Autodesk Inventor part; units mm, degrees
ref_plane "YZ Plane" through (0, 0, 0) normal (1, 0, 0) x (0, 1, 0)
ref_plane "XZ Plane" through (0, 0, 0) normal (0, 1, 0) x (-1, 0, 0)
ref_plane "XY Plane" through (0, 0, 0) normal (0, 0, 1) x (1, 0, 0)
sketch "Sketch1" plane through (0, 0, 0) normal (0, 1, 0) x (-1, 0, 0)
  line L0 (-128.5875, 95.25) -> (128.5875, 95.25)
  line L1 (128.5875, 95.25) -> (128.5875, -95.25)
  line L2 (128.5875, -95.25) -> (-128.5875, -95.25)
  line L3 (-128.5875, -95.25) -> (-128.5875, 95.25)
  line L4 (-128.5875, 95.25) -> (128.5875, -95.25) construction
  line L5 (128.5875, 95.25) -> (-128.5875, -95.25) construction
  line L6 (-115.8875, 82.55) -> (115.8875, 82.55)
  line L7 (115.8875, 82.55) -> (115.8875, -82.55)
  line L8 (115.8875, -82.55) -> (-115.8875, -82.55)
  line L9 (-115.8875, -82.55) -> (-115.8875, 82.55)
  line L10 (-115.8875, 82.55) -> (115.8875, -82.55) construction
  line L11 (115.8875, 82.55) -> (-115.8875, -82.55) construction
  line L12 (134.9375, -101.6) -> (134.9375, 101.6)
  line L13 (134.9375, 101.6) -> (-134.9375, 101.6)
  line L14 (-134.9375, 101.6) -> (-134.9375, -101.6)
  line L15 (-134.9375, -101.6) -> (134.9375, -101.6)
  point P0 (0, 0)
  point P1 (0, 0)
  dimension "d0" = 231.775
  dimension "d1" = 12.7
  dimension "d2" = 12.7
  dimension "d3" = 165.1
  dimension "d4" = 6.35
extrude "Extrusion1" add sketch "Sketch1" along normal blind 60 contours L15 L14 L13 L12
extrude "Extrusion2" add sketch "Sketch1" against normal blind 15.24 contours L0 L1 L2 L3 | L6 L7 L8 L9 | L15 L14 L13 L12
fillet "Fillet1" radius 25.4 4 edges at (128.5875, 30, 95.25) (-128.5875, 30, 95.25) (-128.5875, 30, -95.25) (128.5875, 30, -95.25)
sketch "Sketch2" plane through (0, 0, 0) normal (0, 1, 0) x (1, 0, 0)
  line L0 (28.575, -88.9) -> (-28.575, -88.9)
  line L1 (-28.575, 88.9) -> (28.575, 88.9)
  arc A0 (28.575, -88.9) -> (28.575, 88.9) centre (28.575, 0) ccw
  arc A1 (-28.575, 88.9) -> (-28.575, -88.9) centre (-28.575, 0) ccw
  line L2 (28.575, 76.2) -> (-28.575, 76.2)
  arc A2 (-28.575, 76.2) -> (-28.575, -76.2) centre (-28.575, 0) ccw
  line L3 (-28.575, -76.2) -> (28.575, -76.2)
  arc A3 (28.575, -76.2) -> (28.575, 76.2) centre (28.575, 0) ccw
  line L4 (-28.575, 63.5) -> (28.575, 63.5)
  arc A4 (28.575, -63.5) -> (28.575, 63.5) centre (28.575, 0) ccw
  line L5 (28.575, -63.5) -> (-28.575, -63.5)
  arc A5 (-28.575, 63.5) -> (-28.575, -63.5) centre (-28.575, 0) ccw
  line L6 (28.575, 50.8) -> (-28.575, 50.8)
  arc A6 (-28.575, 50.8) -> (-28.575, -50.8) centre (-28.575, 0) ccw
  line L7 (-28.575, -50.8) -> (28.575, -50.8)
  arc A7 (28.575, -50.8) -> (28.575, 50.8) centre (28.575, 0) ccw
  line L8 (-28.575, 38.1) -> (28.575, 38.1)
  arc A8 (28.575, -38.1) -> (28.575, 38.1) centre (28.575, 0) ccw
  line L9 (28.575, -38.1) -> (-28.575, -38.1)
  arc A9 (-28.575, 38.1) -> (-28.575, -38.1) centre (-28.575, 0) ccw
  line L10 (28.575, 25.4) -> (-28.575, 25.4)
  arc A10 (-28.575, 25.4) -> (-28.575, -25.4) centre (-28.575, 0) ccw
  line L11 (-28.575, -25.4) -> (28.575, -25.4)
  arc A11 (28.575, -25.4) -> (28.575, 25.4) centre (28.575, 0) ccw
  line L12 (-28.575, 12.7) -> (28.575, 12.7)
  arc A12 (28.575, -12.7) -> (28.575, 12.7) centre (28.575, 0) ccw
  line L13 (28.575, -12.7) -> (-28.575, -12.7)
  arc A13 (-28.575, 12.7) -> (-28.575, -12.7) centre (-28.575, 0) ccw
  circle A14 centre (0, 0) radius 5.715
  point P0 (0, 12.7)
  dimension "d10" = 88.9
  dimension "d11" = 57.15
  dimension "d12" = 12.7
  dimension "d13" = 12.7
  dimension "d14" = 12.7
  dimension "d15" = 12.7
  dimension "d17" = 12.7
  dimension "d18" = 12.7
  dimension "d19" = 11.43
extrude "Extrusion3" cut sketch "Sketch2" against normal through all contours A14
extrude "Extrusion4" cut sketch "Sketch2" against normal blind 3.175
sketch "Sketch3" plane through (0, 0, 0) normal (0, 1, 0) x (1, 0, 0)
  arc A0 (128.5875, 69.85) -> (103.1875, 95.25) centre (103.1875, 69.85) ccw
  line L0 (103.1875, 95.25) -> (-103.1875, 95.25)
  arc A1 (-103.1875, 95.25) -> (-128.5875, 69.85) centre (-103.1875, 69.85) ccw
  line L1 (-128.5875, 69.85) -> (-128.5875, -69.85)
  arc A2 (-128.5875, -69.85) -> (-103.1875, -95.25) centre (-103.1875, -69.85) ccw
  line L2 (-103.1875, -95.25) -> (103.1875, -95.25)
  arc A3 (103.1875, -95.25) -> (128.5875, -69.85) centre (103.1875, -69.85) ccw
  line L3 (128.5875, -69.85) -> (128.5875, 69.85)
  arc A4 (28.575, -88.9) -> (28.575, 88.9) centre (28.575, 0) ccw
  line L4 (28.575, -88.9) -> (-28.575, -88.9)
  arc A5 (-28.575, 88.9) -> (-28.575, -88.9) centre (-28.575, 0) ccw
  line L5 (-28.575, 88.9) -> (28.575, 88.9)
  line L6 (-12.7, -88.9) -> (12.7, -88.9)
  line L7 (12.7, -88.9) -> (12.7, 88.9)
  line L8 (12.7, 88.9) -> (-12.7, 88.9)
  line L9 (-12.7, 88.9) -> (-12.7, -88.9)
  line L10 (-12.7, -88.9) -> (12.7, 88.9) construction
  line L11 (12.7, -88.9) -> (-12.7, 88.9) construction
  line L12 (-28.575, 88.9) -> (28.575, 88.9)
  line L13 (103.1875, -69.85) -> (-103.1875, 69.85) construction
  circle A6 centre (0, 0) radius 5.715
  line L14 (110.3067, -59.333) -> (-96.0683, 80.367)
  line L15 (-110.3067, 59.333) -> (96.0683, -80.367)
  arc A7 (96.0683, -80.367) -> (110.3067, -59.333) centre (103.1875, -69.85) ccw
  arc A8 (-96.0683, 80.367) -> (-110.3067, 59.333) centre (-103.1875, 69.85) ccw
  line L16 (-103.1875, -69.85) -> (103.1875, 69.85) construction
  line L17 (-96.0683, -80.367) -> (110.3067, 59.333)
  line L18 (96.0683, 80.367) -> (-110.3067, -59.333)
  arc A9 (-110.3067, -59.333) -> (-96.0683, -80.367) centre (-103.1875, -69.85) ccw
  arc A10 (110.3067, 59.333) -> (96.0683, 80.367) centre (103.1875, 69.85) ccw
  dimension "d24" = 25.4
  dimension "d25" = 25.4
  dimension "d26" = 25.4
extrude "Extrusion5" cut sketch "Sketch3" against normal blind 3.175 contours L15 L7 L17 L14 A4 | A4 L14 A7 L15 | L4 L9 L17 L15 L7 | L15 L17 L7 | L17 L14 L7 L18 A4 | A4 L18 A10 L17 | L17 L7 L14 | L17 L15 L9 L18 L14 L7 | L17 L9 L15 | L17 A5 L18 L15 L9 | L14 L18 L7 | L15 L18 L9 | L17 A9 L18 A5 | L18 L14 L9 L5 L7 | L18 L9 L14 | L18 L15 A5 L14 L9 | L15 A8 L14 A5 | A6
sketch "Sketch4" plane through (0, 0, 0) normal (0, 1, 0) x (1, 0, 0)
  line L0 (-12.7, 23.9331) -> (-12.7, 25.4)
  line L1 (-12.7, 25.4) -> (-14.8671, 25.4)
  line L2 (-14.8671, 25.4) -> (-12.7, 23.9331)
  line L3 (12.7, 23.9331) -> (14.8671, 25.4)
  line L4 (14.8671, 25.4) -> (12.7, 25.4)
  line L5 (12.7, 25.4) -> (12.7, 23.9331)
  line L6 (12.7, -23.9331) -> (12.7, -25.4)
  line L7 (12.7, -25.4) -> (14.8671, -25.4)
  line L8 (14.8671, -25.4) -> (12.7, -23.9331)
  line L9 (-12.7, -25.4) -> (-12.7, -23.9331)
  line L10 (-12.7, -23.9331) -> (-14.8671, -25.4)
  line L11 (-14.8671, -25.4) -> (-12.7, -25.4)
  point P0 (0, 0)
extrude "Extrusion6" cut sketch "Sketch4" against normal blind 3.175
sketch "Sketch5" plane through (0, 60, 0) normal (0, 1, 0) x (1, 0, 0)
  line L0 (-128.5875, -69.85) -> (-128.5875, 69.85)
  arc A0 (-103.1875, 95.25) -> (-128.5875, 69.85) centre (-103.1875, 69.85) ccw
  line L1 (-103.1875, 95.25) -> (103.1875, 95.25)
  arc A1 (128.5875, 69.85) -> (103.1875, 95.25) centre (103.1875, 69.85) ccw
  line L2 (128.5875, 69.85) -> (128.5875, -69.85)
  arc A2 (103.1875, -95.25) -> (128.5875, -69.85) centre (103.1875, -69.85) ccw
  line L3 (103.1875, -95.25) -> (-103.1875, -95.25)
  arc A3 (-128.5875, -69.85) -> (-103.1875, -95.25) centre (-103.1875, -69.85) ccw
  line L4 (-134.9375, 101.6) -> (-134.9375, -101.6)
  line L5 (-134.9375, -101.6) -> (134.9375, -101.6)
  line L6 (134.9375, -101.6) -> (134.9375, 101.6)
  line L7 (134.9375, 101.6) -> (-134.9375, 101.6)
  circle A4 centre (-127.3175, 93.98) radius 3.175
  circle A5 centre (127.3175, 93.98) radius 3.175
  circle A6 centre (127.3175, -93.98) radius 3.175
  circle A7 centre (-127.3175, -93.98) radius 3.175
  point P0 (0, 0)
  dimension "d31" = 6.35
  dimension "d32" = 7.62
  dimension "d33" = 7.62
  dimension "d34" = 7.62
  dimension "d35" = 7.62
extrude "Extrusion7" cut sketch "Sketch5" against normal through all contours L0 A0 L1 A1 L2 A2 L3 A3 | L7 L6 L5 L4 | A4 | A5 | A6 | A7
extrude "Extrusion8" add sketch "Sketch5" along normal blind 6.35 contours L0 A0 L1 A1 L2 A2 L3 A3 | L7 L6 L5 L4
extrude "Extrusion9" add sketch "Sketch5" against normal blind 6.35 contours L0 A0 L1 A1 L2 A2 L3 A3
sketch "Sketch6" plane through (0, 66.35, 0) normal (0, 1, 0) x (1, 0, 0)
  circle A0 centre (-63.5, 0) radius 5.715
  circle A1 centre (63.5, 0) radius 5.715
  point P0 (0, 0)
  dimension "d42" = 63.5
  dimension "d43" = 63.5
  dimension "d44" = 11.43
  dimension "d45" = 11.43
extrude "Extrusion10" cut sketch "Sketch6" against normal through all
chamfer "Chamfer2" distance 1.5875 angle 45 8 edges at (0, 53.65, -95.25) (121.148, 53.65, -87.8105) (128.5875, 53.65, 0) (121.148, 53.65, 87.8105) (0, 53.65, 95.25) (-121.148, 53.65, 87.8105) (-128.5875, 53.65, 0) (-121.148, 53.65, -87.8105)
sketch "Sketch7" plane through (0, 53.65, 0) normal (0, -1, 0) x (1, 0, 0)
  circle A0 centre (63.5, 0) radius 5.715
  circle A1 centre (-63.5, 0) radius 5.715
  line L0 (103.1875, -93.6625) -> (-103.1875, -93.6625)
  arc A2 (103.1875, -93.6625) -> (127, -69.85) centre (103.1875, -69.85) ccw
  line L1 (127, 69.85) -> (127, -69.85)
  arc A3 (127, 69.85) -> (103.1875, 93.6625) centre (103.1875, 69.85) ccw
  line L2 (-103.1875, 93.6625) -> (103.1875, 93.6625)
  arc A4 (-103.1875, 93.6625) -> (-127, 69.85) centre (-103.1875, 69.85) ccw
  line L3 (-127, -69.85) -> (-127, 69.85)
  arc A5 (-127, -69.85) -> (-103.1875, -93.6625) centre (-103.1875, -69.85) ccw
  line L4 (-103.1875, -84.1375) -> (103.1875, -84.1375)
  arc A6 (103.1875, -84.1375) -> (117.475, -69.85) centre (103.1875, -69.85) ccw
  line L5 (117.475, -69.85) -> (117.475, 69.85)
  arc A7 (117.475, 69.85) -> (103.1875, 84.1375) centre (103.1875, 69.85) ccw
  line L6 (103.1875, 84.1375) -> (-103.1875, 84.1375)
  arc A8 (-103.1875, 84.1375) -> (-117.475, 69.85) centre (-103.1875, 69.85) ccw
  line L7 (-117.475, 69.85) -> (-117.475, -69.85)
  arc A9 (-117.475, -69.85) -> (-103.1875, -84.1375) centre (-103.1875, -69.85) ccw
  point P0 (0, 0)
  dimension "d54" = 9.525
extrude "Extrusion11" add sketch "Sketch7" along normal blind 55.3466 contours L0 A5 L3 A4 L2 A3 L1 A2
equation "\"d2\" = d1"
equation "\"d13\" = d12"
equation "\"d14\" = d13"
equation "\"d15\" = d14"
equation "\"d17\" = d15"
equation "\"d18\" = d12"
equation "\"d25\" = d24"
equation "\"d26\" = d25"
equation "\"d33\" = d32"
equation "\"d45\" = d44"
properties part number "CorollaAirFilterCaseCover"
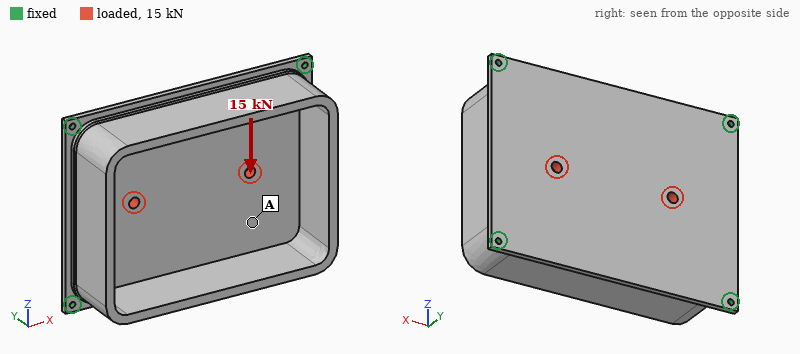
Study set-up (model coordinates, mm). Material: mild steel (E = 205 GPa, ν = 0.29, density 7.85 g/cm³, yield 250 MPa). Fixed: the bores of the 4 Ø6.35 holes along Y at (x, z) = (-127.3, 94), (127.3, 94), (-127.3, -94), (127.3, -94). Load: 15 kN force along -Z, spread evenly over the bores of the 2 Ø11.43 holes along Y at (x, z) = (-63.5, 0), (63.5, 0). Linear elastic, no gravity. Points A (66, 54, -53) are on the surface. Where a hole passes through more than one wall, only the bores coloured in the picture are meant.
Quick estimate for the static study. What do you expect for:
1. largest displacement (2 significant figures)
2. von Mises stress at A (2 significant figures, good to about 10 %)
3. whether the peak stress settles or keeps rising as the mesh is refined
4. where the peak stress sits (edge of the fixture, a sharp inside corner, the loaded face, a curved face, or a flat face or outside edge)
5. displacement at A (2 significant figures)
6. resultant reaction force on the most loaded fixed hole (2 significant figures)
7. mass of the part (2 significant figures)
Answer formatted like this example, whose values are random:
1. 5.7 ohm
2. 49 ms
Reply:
1. 7.6 µm
2. 3.9 MPa
3. keeps rising
4. edge of the fixture
5. 5.7 µm
6. 4.1 kN
7. 8.5 kg
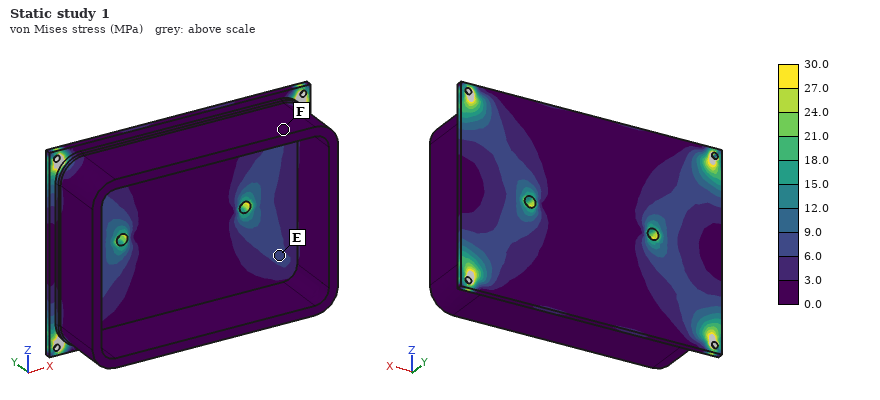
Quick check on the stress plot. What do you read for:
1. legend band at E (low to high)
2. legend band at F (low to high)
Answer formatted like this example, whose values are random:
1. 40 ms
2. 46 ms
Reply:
1. 6.0 to 9.0 MPa
2. 0.0 to 3.0 MPa
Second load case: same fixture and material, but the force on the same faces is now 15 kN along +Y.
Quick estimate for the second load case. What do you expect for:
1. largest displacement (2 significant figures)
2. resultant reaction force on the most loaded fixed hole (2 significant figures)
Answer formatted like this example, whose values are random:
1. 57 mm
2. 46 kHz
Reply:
1. 96 µm
2. 5.1 kN
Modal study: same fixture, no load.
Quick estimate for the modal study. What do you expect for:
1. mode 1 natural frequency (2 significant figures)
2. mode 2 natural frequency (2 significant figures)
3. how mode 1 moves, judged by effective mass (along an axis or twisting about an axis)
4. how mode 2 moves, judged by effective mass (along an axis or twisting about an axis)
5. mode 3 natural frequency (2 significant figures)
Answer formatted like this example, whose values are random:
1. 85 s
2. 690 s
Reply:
1. 1300 Hz
2. 1900 Hz
3. along Y
4. along Z
5. 2000 Hz
